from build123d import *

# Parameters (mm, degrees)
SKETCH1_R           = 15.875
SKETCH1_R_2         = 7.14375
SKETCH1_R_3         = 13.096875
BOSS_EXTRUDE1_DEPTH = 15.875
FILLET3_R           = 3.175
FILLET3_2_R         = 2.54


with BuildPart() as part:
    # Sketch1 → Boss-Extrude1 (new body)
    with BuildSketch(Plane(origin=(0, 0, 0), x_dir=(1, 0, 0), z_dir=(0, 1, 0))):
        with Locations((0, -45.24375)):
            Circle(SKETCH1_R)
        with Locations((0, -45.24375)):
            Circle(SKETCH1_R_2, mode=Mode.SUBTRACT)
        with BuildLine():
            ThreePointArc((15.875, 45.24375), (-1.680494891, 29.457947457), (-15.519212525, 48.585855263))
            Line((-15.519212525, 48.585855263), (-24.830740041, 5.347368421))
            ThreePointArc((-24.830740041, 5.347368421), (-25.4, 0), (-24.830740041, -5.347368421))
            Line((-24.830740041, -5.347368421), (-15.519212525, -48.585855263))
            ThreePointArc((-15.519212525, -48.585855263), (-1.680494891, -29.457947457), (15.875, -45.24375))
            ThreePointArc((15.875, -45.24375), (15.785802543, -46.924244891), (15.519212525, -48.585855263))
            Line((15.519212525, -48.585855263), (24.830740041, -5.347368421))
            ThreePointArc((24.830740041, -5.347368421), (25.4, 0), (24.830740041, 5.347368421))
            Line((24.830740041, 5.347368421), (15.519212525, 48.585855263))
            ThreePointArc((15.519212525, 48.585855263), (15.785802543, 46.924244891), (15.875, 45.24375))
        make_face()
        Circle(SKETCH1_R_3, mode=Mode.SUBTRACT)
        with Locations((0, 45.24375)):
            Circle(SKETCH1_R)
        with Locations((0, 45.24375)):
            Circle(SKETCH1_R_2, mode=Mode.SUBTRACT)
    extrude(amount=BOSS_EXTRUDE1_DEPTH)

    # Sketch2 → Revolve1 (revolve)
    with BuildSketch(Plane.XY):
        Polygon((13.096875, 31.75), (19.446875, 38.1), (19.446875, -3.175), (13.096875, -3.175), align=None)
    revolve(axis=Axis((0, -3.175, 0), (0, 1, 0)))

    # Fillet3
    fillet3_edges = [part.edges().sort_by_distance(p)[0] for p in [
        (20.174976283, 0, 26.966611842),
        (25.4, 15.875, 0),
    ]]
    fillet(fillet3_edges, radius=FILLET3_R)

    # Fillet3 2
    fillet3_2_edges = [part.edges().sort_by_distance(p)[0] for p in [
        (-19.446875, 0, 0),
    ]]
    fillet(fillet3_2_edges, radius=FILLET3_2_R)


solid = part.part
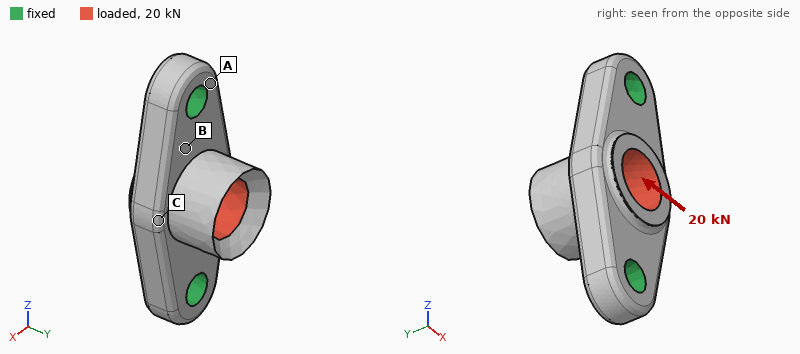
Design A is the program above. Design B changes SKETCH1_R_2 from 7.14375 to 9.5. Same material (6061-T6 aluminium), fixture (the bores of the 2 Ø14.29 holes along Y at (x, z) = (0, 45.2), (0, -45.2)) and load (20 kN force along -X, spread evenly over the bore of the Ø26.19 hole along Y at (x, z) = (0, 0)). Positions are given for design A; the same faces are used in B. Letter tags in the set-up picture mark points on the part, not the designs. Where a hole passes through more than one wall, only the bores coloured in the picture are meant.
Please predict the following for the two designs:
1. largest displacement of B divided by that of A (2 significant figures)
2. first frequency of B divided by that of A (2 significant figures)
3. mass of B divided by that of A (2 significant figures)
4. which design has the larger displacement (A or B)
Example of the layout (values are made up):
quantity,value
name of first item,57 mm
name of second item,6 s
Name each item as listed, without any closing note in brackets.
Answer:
quantity,value
largest displacement of B divided by that of A,0.86
first frequency of B divided by that of A,1.1
mass of B divided by that of A,0.95
which design has the larger displacement,A
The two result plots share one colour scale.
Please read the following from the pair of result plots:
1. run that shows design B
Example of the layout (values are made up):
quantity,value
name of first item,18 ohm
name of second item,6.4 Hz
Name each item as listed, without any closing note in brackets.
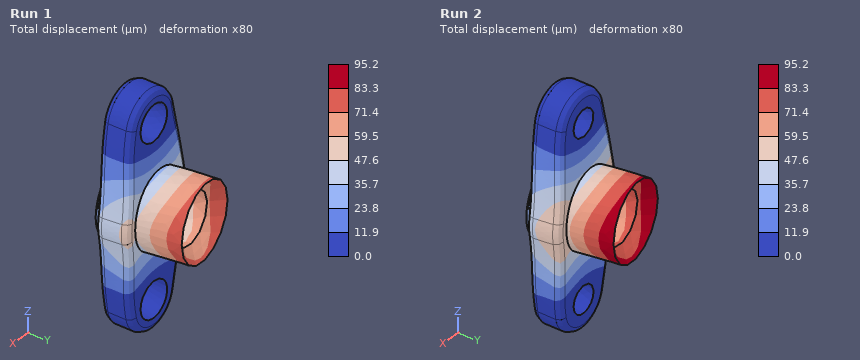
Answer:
quantity,value
run that shows design B,Run 1
